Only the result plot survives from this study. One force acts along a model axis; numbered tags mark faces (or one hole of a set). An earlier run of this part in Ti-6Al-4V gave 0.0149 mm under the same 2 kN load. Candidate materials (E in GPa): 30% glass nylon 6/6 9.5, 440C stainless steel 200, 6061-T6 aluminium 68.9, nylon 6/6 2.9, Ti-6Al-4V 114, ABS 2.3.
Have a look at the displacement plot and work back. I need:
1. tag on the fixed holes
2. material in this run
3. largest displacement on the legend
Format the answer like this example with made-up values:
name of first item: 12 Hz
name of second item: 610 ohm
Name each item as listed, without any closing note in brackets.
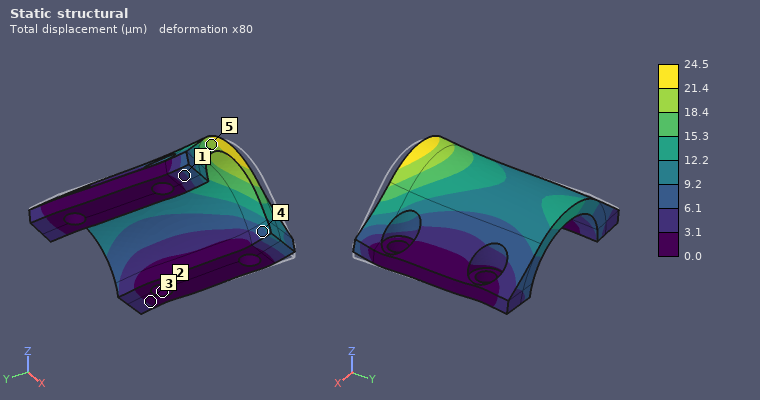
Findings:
tag on the fixed holes: 2
material in this run: 6061-T6 aluminium
largest displacement on the legend: 24.5 µm
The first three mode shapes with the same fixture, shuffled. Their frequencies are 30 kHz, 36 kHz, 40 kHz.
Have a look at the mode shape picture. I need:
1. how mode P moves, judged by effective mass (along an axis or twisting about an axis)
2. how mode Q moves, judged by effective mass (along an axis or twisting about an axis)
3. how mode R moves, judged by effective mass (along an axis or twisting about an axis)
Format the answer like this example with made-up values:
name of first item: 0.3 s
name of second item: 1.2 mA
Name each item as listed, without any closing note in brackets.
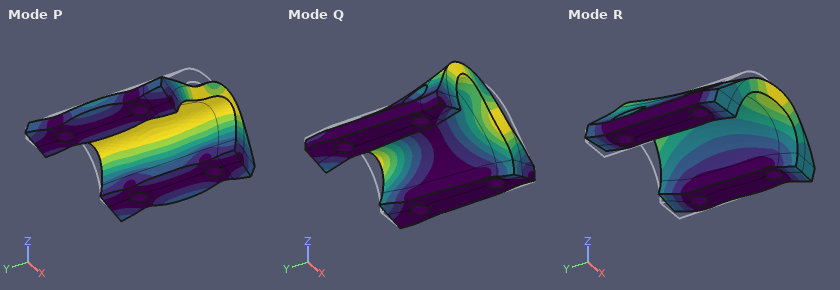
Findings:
how mode P moves, judged by effective mass: along X
how mode Q moves, judged by effective mass: twisting about Z
how mode R moves, judged by effective mass: along Y
